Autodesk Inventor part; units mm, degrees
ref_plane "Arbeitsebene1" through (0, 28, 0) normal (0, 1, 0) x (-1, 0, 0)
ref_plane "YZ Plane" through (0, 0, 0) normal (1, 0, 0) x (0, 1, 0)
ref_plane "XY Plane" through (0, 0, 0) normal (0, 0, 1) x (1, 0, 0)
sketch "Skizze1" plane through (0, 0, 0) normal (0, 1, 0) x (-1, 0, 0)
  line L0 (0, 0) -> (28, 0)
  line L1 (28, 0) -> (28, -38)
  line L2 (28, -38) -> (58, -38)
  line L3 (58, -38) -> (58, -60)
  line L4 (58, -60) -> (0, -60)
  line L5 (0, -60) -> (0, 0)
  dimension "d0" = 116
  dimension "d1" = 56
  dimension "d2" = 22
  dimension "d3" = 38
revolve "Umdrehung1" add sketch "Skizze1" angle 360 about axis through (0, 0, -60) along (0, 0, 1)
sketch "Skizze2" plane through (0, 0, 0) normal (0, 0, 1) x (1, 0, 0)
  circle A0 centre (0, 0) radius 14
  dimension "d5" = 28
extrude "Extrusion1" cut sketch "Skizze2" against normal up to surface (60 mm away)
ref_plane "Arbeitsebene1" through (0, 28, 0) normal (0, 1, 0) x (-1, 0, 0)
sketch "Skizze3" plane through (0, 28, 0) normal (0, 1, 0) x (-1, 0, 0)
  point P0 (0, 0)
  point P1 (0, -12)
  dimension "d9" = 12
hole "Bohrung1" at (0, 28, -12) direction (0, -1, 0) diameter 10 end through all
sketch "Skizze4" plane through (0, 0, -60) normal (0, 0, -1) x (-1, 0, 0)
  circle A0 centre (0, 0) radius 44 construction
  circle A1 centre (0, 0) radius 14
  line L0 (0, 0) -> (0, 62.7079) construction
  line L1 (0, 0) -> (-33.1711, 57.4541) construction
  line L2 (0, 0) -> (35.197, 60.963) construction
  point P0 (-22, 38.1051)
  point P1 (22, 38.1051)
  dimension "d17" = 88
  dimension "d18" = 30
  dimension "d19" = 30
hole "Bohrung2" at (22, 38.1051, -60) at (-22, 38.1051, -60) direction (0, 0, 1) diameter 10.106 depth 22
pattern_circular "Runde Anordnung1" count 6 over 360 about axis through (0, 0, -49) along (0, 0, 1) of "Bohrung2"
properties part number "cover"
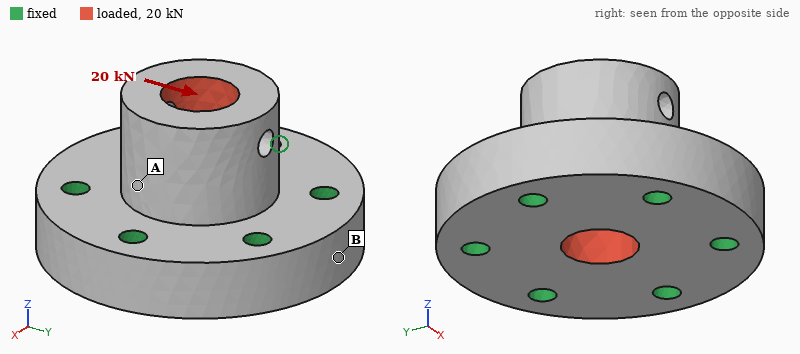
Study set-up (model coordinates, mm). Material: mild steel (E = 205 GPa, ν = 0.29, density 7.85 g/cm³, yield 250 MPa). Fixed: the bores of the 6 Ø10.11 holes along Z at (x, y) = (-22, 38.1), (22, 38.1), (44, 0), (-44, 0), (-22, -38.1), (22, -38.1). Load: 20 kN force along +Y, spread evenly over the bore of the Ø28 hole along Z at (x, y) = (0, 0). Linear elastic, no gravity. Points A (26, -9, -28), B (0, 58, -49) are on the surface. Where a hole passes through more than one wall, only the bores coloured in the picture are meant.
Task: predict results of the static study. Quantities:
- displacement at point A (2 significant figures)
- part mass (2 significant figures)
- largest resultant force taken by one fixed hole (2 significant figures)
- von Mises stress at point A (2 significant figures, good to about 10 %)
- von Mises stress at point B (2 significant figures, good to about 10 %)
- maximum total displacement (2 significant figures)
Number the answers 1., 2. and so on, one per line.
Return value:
1. 2.8 µm
2. 2.2 kg
3. 5.1 kN
4. 9.2 MPa
5. 3.3 MPa
6. 7.3 µm
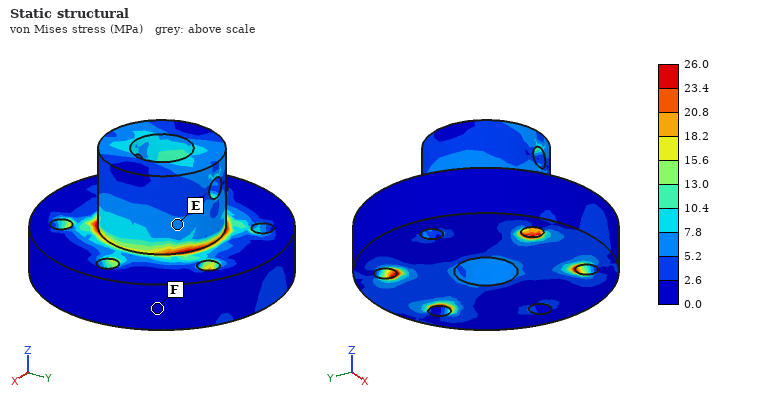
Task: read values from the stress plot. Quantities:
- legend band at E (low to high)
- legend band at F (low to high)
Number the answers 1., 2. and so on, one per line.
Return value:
1. 5.2 to 7.8 MPa
2. 0.0 to 2.6 MPa
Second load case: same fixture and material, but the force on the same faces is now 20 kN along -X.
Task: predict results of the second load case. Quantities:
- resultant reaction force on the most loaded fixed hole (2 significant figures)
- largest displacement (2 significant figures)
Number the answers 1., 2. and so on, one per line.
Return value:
1. 5.8 kN
2. 7.7 µm
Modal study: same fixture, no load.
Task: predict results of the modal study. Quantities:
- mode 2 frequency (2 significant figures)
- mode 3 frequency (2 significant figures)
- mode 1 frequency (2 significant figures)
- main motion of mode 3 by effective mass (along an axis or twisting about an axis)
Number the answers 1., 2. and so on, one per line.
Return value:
1. 11 kHz
2. 15 kHz
3. 10 kHz
4. along Z
